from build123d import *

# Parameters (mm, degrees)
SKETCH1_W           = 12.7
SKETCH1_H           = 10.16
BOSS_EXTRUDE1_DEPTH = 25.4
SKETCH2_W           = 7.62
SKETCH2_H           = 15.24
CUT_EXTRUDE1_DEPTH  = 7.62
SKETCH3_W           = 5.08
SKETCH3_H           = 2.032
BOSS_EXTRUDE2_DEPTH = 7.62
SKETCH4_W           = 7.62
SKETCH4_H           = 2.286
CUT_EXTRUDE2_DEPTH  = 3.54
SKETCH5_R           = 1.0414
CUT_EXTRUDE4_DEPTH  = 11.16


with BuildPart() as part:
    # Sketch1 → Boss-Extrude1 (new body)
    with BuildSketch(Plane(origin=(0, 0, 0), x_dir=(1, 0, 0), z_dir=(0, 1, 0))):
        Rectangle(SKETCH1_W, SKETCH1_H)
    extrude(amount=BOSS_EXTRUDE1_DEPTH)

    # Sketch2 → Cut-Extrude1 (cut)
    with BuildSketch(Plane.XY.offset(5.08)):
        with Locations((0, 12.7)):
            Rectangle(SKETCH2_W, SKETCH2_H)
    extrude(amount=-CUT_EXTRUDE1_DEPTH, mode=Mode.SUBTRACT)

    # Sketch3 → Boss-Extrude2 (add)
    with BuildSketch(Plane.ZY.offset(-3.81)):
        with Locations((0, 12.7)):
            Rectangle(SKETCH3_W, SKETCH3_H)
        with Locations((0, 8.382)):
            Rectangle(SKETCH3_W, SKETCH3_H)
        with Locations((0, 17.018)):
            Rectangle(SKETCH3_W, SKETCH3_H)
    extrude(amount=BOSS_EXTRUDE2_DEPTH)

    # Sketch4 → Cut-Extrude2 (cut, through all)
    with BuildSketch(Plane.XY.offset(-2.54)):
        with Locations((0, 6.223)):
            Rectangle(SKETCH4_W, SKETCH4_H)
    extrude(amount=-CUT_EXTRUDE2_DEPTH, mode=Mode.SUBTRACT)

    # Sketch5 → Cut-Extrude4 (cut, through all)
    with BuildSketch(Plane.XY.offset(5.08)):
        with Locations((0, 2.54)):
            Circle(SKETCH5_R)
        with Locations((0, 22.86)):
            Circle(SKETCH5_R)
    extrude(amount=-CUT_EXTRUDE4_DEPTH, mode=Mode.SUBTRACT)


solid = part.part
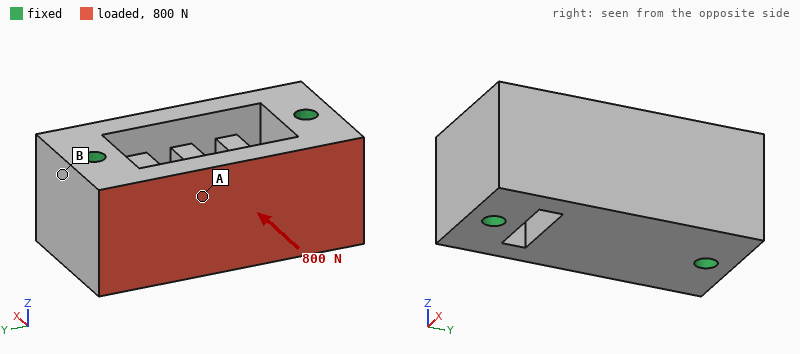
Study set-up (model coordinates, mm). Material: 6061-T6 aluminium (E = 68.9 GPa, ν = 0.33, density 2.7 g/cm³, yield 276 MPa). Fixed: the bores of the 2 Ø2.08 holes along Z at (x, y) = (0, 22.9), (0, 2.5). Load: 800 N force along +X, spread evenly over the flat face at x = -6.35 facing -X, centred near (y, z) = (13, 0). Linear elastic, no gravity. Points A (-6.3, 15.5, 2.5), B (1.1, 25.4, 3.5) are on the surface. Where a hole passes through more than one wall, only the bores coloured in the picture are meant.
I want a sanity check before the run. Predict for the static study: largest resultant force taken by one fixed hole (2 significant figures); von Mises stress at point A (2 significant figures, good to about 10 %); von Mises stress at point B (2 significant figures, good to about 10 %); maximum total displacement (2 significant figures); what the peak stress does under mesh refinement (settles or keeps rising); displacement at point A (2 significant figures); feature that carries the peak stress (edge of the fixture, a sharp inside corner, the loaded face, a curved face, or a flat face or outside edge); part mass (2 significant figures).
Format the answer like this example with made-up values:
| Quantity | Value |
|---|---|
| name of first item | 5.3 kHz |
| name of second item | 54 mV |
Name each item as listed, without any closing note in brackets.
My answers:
| Quantity | Value |
|---|---|
| largest resultant force taken by one fixed hole | 410 N |
| von Mises stress at point A | 11 MPa |
| von Mises stress at point B | 3.1 MPa |
| maximum total displacement | 5.1 µm |
| what the peak stress does under mesh refinement | keeps rising |
| displacement at point A | 3.5 µm |
| feature that carries the peak stress | edge of the fixture |
| part mass | 6.8 g |
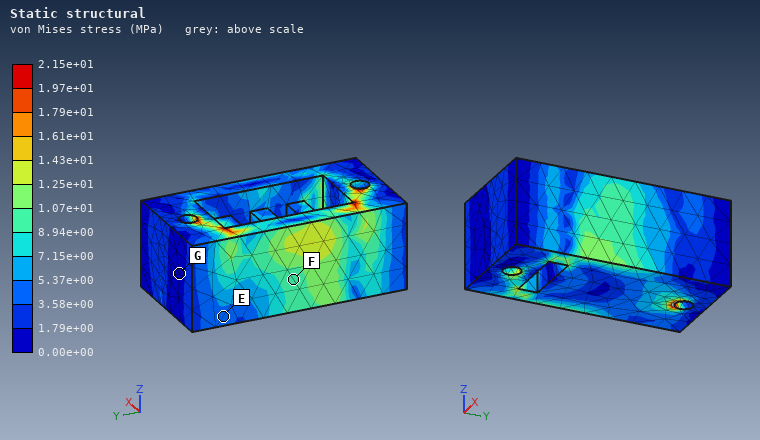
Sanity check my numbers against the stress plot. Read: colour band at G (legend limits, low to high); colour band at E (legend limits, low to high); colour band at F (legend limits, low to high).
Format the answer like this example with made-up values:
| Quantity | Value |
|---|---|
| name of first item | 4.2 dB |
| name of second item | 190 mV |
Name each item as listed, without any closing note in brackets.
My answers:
| Quantity | Value |
|---|---|
| colour band at G | 0.00e+00 to 1.79e+00 MPa |
| colour band at E | 3.58e+00 to 5.37e+00 MPa |
| colour band at F | 8.94e+00 to 1.07e+01 MPa |
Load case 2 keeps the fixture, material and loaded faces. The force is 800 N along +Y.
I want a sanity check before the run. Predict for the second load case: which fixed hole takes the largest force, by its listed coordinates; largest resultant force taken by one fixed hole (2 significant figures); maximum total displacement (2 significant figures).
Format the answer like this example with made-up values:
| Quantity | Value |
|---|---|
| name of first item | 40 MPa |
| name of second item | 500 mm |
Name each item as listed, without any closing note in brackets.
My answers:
| Quantity | Value |
|---|---|
| which fixed hole takes the largest force, by its listed coordinates | (0, 22.9) |
| largest resultant force taken by one fixed hole | 500 N |
| maximum total displacement | 3.5 µm |
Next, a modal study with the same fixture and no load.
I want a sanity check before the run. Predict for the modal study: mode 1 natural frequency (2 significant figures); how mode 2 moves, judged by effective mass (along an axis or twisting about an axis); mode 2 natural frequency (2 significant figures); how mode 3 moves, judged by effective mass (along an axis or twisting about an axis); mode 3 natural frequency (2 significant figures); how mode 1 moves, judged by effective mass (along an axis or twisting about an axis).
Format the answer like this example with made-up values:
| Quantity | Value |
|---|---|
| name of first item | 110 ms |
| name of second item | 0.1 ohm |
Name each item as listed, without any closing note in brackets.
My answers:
| Quantity | Value |
|---|---|
| mode 1 natural frequency | 38 kHz |
| how mode 2 moves, judged by effective mass | along Z |
| mode 2 natural frequency | 42 kHz |
| how mode 3 moves, judged by effective mass | twisting about Y |
| mode 3 natural frequency | 49 kHz |
| how mode 1 moves, judged by effective mass | along X |
